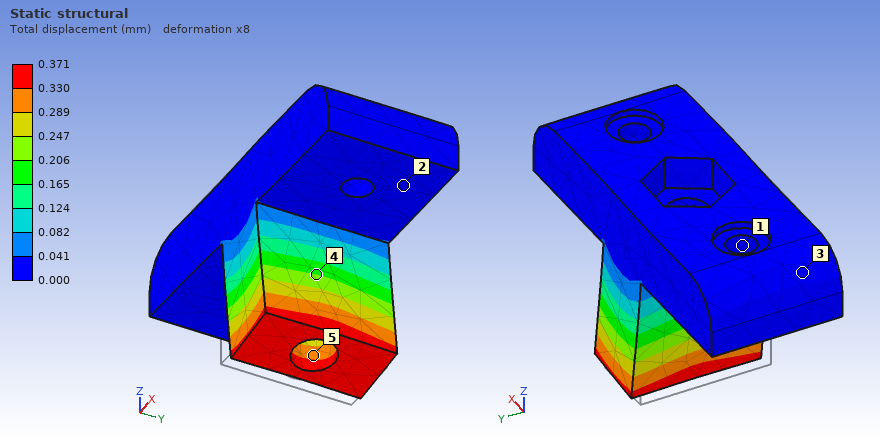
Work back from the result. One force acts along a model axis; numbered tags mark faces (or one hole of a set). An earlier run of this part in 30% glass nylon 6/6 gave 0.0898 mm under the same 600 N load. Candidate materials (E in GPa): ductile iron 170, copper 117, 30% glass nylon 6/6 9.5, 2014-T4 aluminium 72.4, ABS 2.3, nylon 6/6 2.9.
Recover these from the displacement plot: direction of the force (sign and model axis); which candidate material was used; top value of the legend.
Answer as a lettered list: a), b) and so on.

a) +X
b) ABS
c) 0.371 mm
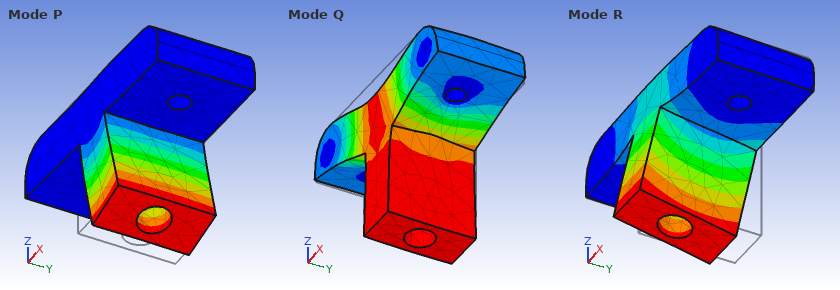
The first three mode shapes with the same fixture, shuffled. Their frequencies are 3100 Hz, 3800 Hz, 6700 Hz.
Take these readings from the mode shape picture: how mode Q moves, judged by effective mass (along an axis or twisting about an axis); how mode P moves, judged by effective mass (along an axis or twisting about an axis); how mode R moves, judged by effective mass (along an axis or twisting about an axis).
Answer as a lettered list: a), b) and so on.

a) along Z
b) along X
c) along Y
